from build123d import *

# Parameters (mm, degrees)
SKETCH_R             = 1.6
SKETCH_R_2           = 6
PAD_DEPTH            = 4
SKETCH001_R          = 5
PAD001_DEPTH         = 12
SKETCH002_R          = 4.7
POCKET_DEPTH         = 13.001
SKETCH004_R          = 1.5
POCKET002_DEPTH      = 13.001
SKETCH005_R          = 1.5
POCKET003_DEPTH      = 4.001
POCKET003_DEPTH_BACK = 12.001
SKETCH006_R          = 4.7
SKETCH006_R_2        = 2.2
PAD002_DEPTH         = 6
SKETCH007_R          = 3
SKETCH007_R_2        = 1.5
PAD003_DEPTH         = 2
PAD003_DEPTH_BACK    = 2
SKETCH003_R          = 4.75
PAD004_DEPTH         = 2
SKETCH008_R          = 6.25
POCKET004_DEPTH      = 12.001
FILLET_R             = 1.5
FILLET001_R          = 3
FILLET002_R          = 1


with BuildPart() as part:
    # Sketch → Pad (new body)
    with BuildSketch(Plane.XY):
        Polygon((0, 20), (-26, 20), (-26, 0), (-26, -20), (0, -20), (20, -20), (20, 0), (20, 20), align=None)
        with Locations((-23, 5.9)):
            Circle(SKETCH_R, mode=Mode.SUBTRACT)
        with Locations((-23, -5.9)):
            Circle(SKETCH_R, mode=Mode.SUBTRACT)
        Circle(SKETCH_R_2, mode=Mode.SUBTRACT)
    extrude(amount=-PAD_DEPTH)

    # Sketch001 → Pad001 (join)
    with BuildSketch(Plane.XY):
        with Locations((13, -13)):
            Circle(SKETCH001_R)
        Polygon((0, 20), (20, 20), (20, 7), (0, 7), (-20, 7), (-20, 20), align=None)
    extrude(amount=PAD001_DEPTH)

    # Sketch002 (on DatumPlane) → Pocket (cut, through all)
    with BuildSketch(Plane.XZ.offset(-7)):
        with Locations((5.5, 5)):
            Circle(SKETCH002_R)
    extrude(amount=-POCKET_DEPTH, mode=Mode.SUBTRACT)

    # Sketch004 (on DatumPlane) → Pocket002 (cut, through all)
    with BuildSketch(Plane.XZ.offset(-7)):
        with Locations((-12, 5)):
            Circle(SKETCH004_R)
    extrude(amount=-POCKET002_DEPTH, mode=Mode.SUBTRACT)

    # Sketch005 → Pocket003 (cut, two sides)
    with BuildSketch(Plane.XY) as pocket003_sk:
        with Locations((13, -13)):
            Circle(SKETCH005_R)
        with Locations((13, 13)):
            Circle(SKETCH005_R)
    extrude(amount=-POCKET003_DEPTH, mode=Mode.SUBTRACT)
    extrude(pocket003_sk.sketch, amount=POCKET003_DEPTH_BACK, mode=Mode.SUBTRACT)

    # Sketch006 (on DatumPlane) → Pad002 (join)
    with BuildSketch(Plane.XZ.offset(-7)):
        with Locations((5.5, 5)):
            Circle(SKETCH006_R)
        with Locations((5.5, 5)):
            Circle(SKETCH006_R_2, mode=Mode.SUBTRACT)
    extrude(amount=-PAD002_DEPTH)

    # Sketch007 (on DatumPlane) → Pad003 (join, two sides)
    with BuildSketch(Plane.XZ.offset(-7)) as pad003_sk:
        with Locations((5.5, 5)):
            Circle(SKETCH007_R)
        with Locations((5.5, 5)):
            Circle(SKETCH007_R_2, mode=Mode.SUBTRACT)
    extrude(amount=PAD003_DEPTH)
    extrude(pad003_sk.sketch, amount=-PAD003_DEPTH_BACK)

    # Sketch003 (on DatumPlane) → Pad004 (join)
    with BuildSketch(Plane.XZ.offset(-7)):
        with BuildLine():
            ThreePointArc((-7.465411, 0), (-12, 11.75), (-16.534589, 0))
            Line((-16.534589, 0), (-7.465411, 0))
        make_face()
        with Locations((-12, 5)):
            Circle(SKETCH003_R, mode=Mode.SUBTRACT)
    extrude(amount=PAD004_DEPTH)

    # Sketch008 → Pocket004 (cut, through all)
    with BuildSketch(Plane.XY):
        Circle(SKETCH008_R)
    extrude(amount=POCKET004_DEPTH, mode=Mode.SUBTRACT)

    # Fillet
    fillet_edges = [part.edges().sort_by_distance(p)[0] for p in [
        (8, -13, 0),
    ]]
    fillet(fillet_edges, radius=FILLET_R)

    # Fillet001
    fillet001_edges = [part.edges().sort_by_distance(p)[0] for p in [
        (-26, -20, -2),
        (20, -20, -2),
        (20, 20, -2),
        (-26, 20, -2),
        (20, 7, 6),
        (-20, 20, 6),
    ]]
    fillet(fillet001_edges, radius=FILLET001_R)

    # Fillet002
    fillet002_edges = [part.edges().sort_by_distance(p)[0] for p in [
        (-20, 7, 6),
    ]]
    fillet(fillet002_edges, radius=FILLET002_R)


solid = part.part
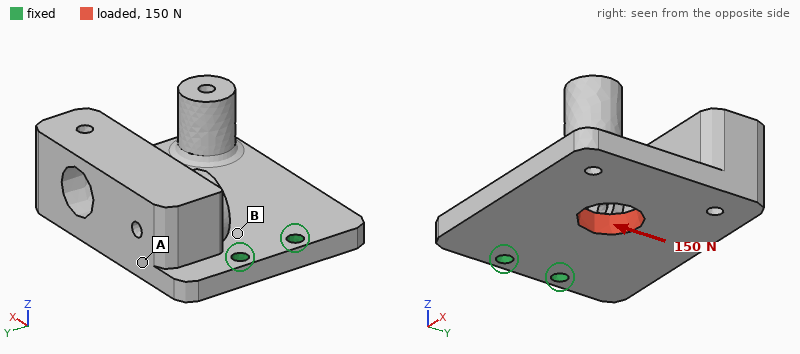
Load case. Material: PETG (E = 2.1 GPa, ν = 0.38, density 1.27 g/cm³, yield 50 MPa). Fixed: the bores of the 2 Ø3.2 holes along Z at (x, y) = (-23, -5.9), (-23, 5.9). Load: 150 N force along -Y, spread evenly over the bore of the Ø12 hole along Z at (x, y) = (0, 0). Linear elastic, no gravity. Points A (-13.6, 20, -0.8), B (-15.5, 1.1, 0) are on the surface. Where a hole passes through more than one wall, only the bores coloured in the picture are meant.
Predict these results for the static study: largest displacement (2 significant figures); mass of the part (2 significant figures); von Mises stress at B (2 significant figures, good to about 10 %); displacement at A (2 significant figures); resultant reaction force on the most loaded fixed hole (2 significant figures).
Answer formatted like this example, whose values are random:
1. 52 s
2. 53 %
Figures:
1. 0.27 mm
2. 17 g
3. 6.3 MPa
4. 0.12 mm
5. 240 N
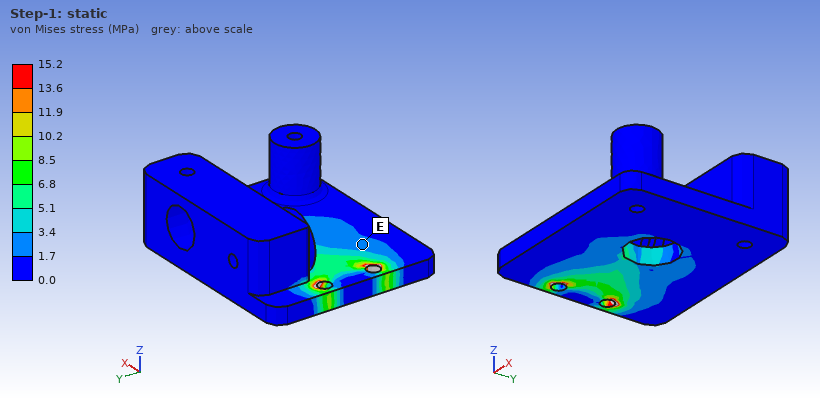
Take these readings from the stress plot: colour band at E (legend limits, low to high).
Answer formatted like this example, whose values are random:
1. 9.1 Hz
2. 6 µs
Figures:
1. 1.7 to 3.4 MPa
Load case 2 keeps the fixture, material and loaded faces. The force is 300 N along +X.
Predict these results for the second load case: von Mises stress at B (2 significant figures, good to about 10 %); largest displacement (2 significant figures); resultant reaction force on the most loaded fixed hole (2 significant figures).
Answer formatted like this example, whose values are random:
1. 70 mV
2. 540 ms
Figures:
1. 2.3 MPa
2. 64 µm
3. 150 N
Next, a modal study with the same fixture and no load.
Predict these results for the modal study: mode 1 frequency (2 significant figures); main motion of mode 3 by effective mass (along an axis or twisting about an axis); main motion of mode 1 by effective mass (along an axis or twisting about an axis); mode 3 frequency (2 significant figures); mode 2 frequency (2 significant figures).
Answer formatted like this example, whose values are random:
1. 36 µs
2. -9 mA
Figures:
1. 330 Hz
2. along Y
3. along Z
4. 1100 Hz
5. 700 Hz
